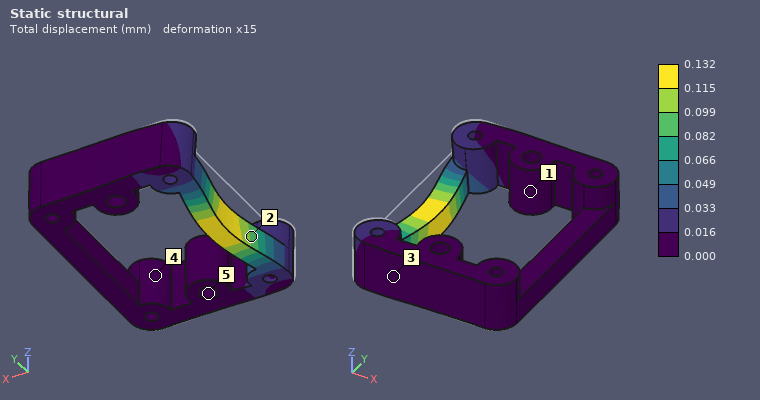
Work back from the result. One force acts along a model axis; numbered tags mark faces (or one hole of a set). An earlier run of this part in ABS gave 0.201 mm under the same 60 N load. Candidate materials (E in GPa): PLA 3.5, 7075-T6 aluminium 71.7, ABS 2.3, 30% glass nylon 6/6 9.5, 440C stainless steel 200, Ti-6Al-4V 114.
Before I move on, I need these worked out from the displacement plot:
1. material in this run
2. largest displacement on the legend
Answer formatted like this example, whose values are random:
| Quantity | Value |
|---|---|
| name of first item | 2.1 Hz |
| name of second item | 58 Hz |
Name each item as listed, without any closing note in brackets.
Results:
| Quantity | Value |
|---|---|
| material in this run | PLA |
| largest displacement on the legend | 0.132 mm |
